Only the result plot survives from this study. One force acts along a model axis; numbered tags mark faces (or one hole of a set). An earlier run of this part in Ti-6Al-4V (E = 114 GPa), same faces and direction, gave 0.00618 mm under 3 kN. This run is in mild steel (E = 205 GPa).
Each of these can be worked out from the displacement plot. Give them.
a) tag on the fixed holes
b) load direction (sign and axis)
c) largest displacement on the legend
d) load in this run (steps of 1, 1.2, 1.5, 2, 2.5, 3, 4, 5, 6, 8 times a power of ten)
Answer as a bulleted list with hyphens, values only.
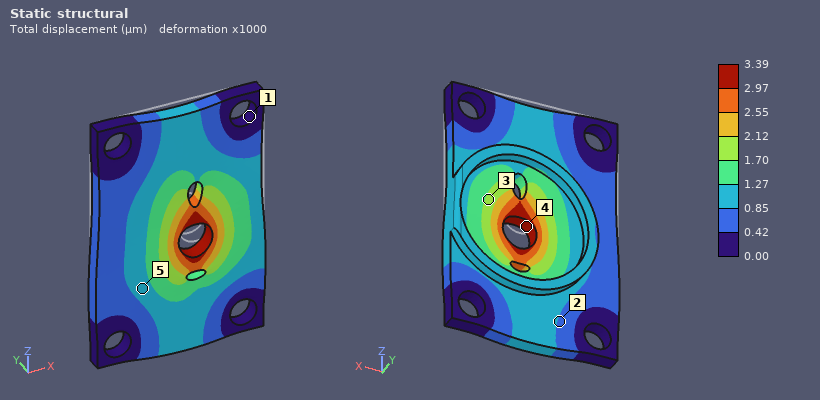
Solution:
- 1
- -Z
- 3.39 µm
- 3 kN
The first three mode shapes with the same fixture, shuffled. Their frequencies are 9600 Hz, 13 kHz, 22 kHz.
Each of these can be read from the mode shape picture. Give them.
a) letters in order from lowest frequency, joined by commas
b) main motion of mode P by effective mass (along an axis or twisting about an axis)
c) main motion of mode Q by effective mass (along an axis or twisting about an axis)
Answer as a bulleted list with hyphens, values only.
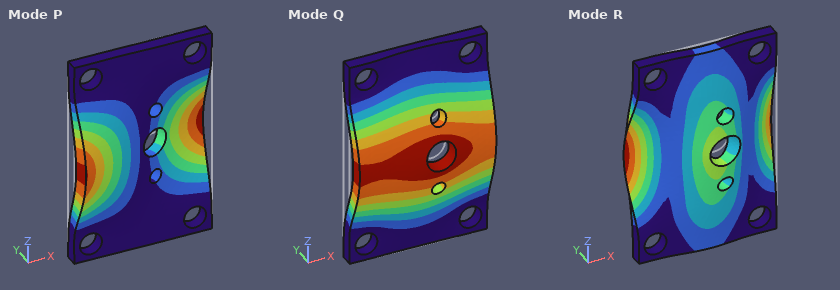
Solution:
- Q, P, R
- twisting about Z
- along Y
